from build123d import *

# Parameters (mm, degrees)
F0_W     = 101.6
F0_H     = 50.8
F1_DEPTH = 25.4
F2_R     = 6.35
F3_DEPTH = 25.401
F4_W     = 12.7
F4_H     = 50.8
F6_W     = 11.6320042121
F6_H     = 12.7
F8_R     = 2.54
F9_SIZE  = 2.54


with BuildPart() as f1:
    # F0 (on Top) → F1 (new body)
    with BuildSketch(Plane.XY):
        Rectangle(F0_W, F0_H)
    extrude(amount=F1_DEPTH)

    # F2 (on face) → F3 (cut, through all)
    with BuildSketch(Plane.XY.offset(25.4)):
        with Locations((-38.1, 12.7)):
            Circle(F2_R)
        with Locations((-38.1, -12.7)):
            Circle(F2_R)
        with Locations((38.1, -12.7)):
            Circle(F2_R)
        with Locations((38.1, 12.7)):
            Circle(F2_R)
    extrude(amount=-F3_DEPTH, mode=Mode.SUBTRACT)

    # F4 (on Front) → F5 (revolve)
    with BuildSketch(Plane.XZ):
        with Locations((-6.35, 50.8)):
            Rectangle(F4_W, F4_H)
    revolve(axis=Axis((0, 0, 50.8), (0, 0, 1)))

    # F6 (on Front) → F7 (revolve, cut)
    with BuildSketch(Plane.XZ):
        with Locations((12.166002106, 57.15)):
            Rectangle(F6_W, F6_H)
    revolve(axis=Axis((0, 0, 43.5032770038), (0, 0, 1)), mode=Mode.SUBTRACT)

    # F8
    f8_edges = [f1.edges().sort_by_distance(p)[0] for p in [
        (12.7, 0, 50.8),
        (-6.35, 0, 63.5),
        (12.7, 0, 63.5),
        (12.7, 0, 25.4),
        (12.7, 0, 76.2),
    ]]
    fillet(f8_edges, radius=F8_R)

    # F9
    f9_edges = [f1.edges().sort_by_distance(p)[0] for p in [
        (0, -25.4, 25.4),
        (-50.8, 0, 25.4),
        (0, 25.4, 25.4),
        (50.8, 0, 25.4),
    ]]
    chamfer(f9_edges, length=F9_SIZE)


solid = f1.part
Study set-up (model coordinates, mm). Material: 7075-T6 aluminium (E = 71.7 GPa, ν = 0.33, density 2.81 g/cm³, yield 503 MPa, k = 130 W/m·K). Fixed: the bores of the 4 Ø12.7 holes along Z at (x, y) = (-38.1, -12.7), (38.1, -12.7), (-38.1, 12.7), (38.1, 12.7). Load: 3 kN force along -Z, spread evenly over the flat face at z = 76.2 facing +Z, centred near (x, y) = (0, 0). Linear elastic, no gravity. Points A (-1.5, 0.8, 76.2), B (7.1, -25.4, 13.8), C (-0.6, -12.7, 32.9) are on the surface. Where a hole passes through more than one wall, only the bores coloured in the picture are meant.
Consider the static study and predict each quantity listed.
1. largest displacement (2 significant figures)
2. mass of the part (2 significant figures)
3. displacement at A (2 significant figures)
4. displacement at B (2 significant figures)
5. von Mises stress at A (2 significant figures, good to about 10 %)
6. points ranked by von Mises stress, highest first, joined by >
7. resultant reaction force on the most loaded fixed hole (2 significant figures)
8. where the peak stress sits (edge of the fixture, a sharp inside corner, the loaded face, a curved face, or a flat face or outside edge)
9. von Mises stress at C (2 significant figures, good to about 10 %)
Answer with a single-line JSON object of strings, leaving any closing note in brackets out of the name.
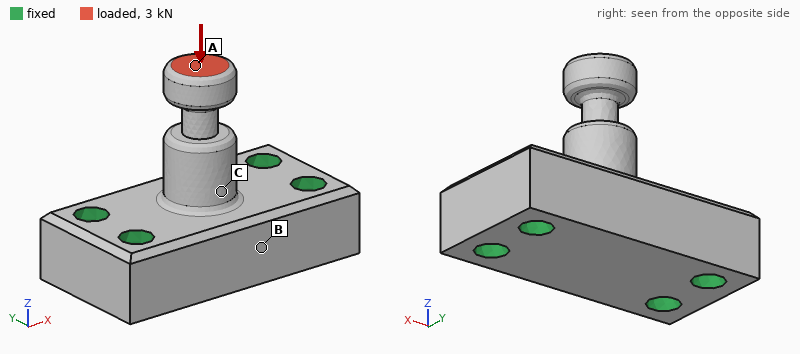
{"largest displacement": "11 µm", "mass of the part": "390 g", "displacement at A": "11 µm", "displacement at B": "1.7 µm", "von Mises stress at A": "9.1 MPa", "points ranked by von Mises stress, highest first, joined by >": "A > C > B", "resultant reaction force on the most loaded fixed hole": "770 N", "where the peak stress sits": "a curved face", "von Mises stress at C": "5.4 MPa"}
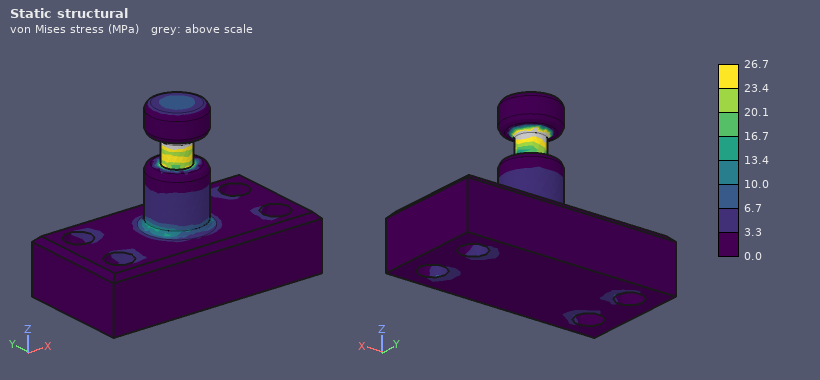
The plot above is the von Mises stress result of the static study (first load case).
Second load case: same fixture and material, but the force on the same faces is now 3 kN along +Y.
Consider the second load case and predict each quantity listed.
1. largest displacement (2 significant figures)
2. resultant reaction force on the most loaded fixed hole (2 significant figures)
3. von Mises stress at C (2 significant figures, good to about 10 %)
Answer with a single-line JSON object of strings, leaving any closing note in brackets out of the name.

{"largest displacement": "0.38 mm", "resultant reaction force on the most loaded fixed hole": "2.5 kN", "von Mises stress at C": "78 MPa"}
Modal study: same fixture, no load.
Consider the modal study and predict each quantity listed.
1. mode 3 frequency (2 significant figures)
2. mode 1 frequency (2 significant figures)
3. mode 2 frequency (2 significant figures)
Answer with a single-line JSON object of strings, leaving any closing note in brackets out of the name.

{"mode 3 frequency": "8600 Hz", "mode 1 frequency": "4100 Hz", "mode 2 frequency": "4300 Hz"}
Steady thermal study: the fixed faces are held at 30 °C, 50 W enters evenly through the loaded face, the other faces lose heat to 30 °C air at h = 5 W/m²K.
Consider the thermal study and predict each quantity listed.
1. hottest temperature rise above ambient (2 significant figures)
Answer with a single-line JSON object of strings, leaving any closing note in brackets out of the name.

{"hottest temperature rise above ambient": "85 K"}
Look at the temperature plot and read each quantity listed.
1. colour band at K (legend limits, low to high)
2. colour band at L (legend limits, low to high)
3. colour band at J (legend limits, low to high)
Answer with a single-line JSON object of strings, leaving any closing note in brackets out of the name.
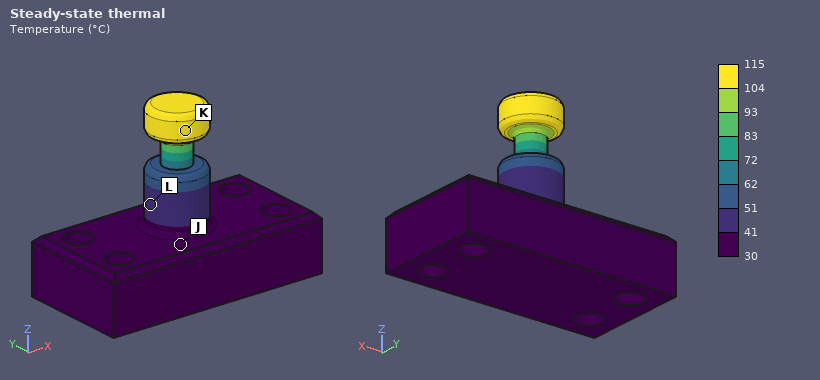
{"colour band at K": "104 to 115 °C", "colour band at L": "41 to 51 °C", "colour band at J": "30 to 41 °C"}
